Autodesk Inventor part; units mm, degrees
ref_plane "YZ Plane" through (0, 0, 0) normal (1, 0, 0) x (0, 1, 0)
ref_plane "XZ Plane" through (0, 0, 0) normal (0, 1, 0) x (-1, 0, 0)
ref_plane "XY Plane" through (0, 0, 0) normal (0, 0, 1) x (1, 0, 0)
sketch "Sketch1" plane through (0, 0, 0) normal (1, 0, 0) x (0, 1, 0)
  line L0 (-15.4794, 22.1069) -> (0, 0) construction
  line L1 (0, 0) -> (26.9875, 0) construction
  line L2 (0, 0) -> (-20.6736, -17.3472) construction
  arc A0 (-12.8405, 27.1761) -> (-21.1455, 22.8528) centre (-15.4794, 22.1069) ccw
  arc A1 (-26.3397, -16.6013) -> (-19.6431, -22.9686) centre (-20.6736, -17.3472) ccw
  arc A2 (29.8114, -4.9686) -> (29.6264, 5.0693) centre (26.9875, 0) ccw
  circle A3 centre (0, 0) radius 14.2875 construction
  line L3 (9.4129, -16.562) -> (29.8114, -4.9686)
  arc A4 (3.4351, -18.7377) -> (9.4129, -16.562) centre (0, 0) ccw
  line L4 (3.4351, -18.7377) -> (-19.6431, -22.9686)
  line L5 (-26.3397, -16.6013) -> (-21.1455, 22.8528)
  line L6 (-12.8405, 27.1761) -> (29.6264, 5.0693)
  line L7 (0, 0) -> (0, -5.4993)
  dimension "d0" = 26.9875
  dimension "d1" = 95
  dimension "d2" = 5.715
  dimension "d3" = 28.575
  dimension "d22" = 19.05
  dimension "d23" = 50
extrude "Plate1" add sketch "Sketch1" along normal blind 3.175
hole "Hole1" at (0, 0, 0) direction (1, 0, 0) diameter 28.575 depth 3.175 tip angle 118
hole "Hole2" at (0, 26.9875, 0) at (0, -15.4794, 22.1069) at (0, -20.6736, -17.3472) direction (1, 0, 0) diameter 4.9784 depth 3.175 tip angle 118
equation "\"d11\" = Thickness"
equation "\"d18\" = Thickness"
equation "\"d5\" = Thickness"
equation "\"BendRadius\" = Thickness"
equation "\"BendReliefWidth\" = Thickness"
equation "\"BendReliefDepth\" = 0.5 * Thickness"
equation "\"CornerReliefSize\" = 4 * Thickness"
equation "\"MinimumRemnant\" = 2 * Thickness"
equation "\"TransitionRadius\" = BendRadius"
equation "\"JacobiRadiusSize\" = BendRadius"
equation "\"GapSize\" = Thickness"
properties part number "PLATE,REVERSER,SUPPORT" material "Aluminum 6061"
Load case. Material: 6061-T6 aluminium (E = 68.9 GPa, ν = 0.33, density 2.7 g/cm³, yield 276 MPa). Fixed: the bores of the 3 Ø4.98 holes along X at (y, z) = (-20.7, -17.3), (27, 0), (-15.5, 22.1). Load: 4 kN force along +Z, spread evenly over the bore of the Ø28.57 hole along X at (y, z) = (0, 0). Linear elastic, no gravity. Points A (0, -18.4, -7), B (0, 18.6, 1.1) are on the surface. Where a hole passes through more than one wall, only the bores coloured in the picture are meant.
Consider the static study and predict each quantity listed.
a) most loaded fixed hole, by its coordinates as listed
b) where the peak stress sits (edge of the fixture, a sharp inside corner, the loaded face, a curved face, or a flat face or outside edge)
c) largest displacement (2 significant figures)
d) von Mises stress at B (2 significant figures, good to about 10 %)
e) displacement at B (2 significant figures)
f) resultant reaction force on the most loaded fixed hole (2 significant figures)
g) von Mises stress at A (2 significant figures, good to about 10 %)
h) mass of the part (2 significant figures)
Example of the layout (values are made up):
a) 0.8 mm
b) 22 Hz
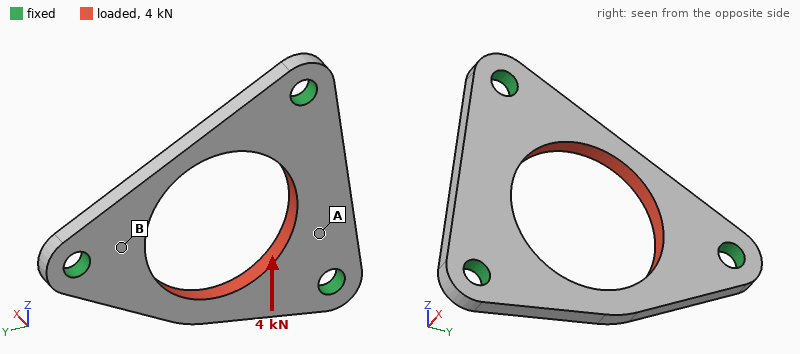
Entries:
a) (27, 0)
b) edge of the fixture
c) 50 µm
d) 58 MPa
e) 22 µm
f) 1.8 kN
g) 25 MPa
h) 10 g
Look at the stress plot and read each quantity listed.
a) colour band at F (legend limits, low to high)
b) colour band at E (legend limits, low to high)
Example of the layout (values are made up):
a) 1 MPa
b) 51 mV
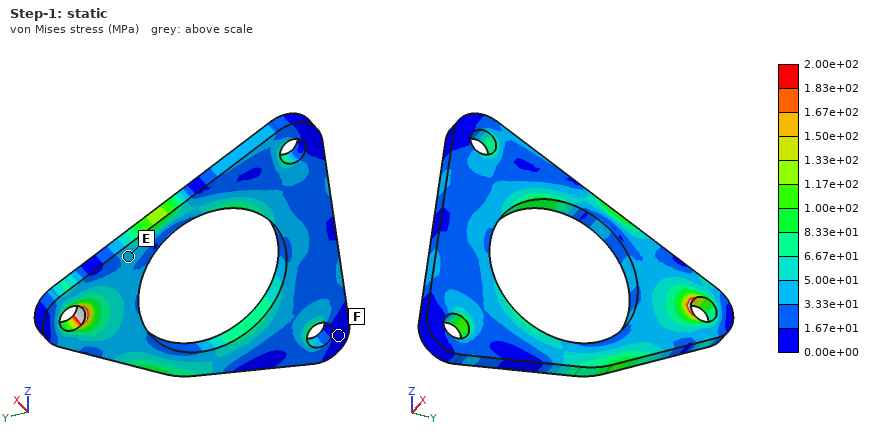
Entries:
a) 0.00e+00 to 1.67e+01 MPa
b) 3.33e+01 to 5.00e+01 MPa
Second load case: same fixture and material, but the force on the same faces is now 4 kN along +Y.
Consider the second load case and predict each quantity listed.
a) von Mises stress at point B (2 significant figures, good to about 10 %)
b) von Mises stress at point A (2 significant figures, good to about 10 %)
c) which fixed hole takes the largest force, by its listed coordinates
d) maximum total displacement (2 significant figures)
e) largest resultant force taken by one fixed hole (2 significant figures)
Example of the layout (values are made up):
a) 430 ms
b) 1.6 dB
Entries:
a) 21 MPa
b) 30 MPa
c) (-20.7, -17.3)
d) 25 µm
e) 1.6 kN
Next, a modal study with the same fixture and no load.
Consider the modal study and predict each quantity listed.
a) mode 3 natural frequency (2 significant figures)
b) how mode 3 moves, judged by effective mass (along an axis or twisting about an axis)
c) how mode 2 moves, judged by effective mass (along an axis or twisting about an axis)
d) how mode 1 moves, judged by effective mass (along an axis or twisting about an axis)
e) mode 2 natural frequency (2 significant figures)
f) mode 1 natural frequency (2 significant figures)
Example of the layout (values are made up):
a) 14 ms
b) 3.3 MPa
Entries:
a) 12 kHz
b) along X
c) along X
d) along X
e) 10000 Hz
f) 8000 Hz
